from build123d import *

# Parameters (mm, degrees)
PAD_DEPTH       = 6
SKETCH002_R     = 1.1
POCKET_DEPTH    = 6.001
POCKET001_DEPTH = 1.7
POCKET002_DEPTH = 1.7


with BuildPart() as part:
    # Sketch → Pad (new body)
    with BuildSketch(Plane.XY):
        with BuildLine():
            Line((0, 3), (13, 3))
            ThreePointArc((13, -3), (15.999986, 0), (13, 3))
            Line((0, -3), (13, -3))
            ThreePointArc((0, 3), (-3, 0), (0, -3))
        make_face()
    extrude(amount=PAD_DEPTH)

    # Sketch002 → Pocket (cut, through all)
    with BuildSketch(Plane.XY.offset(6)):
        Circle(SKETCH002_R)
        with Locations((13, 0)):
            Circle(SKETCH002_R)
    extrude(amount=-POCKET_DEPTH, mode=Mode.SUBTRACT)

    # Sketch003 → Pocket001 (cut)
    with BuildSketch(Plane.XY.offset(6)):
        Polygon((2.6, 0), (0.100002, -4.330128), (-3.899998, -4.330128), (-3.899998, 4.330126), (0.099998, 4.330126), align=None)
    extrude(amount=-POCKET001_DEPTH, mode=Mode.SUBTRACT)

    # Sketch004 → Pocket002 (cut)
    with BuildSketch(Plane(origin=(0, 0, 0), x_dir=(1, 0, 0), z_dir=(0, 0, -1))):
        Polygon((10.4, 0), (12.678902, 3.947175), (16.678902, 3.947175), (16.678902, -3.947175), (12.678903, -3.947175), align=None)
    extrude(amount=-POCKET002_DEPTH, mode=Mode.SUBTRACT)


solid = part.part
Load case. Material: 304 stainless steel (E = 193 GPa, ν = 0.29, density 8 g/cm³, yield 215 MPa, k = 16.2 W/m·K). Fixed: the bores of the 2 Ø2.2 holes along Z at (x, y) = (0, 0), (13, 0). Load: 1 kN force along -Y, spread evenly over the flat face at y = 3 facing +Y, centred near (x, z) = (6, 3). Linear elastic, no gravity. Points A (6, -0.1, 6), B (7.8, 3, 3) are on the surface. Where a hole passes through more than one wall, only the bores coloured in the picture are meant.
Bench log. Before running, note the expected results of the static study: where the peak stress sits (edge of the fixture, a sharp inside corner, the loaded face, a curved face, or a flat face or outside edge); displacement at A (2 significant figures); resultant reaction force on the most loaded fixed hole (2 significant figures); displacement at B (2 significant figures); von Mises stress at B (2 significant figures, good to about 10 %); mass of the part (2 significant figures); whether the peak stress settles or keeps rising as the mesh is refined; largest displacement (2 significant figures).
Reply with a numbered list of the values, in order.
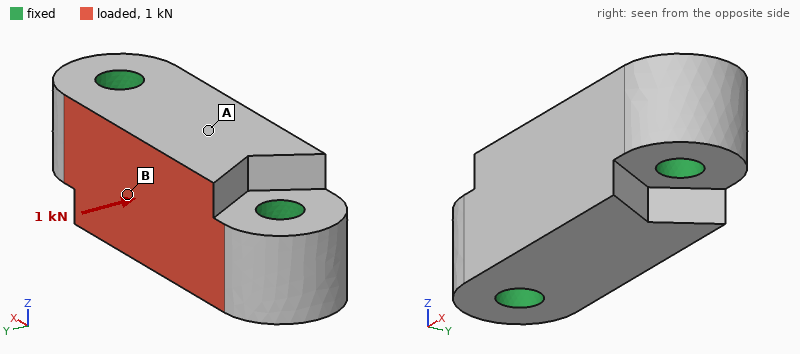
1. edge of the fixture
2. 1.4 µm
3. 500 N
4. 1.3 µm
5. 28 MPa
6. 4.2 g
7. keeps rising
8. 1.6 µm
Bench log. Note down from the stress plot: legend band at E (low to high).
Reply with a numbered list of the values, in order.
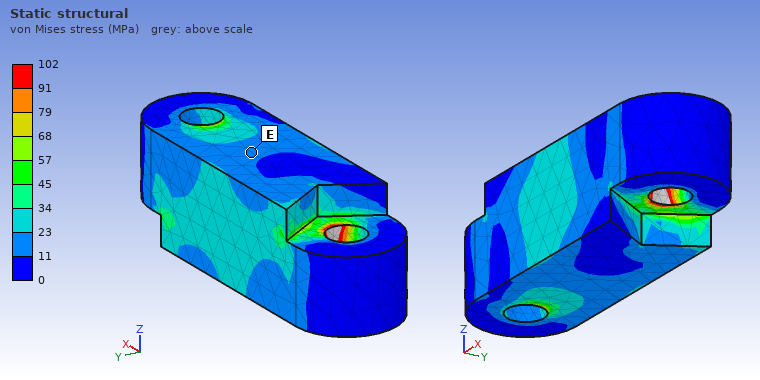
1. 11 to 23 MPa
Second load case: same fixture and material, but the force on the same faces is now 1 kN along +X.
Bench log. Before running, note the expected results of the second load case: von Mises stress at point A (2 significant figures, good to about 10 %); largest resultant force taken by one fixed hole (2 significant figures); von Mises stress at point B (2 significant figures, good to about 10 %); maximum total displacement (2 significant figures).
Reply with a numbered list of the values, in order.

1. 9.6 MPa
2. 540 N
3. 24 MPa
4. 1.9 µm
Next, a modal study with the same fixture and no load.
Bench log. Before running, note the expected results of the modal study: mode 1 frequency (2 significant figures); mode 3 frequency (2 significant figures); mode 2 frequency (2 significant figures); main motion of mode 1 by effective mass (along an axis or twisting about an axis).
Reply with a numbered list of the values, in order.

1. 80 kHz
2. 86 kHz
3. 85 kHz
4. along Y
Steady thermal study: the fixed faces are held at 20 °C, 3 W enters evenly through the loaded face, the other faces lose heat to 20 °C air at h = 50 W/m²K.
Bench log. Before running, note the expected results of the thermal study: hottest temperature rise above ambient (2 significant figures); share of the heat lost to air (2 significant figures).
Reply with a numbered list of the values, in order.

1. 15 K
2. 3.0 %
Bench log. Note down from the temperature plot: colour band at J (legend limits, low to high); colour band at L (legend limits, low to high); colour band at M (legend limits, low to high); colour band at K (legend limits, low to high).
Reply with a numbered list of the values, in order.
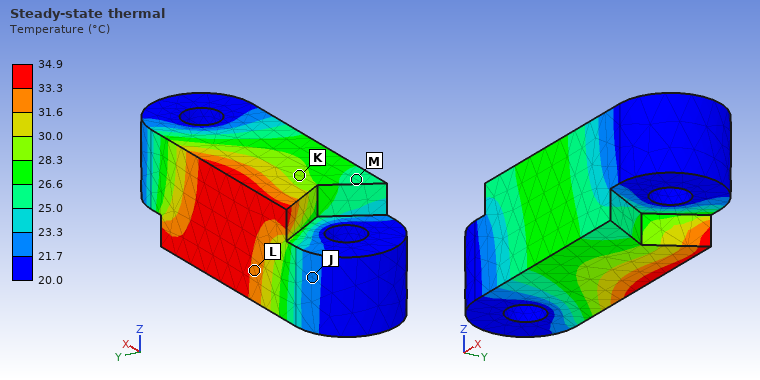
1. 21.7 to 23.3 °C
2. 31.6 to 33.3 °C
3. 25.0 to 26.6 °C
4. 28.3 to 30.0 °C
